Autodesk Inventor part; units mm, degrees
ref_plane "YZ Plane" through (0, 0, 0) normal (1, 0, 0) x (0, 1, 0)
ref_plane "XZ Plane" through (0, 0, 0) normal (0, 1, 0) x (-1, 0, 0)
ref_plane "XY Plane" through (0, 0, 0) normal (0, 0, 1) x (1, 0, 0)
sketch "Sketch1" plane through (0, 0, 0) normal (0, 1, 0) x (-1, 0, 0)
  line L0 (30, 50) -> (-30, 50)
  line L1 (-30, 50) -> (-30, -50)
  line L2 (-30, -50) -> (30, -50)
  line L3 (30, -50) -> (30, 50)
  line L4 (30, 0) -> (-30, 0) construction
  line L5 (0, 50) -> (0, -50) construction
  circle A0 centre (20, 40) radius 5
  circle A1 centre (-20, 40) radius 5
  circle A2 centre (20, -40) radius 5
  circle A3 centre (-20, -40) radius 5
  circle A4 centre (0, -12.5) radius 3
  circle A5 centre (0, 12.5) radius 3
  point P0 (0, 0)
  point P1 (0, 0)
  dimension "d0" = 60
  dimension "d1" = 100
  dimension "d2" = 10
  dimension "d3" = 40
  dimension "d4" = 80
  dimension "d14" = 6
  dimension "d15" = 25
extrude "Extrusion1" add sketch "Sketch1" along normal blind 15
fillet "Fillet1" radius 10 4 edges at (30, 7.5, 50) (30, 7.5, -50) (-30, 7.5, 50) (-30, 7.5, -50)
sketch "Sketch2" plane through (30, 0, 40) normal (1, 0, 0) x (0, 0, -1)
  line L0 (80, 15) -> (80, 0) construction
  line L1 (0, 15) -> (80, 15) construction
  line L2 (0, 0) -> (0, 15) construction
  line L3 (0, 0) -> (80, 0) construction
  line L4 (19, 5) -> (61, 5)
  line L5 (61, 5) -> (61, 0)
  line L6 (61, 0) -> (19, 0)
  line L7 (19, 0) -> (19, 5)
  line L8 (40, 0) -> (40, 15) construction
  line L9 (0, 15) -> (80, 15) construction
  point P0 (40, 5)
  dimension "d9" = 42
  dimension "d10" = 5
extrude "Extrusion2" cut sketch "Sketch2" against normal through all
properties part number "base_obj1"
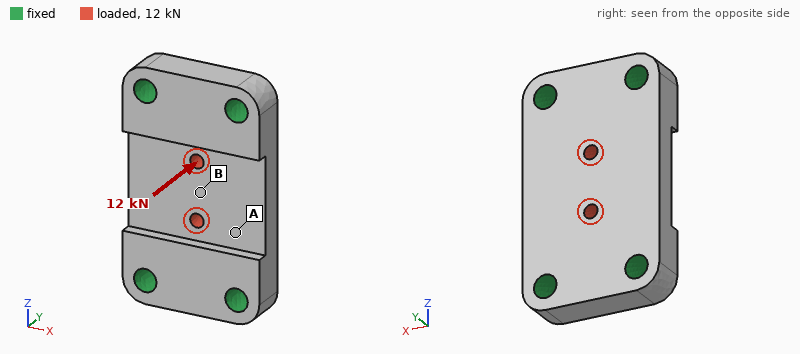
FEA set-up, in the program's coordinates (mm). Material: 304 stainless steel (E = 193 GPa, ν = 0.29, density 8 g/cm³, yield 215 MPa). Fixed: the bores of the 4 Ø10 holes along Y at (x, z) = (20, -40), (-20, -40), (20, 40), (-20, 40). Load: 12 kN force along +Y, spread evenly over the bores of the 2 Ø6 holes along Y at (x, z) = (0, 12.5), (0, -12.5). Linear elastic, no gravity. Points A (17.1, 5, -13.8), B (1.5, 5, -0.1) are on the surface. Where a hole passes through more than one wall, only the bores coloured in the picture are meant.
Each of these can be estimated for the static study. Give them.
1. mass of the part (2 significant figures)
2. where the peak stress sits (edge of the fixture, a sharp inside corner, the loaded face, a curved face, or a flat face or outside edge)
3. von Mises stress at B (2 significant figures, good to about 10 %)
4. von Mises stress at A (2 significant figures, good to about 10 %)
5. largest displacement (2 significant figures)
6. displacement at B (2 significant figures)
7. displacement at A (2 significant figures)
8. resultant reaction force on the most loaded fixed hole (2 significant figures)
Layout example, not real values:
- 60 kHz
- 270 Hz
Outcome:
- 570 g
- the loaded face
- 55 MPa
- 21 MPa
- 21 µm
- 20 µm
- 10 µm
- 3.4 kN
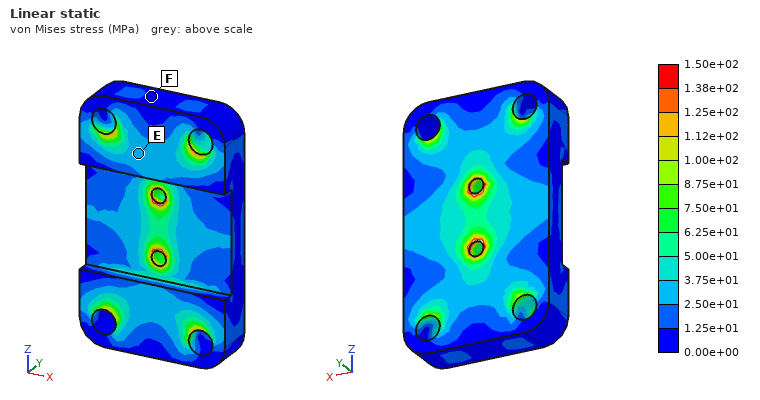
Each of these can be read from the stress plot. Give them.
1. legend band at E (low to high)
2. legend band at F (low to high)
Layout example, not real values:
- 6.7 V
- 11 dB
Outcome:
- 2.50e+01 to 3.75e+01 MPa
- 0.00e+00 to 1.25e+01 MPa
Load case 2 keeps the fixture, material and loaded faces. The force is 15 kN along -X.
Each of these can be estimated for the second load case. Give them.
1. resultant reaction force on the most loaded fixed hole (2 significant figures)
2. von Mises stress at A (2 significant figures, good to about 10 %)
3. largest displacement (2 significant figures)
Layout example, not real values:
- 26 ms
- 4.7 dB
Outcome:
- 4.9 kN
- 17 MPa
- 6.2 µm
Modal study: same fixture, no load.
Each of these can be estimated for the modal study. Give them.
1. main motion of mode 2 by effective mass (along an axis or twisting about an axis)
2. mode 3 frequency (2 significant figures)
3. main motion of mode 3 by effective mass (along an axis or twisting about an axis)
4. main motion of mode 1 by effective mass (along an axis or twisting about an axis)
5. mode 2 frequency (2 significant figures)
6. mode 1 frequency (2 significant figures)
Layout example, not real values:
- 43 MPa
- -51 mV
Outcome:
- twisting about Z
- 19 kHz
- along X
- along Y
- 13 kHz
- 10 kHz
